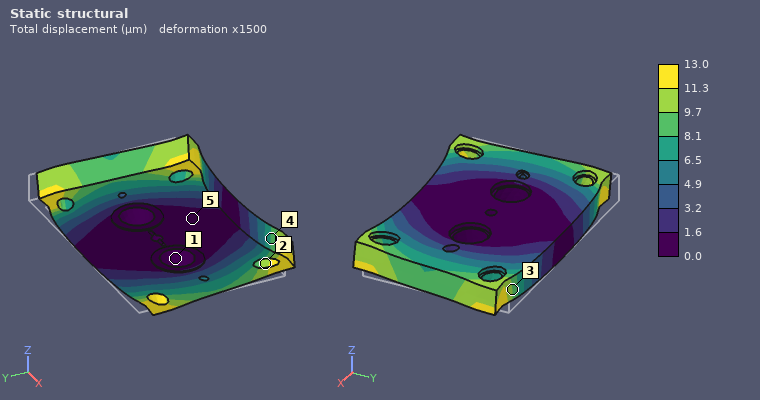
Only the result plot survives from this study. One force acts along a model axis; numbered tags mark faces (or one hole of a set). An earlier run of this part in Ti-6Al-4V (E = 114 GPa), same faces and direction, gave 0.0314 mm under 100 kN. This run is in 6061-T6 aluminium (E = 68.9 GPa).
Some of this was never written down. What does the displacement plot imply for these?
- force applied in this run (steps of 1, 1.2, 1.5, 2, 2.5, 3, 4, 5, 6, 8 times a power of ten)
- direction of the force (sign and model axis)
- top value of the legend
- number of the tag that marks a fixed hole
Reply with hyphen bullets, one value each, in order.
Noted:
- 25 kN
- -Y
- 13.0 µm
- 1
